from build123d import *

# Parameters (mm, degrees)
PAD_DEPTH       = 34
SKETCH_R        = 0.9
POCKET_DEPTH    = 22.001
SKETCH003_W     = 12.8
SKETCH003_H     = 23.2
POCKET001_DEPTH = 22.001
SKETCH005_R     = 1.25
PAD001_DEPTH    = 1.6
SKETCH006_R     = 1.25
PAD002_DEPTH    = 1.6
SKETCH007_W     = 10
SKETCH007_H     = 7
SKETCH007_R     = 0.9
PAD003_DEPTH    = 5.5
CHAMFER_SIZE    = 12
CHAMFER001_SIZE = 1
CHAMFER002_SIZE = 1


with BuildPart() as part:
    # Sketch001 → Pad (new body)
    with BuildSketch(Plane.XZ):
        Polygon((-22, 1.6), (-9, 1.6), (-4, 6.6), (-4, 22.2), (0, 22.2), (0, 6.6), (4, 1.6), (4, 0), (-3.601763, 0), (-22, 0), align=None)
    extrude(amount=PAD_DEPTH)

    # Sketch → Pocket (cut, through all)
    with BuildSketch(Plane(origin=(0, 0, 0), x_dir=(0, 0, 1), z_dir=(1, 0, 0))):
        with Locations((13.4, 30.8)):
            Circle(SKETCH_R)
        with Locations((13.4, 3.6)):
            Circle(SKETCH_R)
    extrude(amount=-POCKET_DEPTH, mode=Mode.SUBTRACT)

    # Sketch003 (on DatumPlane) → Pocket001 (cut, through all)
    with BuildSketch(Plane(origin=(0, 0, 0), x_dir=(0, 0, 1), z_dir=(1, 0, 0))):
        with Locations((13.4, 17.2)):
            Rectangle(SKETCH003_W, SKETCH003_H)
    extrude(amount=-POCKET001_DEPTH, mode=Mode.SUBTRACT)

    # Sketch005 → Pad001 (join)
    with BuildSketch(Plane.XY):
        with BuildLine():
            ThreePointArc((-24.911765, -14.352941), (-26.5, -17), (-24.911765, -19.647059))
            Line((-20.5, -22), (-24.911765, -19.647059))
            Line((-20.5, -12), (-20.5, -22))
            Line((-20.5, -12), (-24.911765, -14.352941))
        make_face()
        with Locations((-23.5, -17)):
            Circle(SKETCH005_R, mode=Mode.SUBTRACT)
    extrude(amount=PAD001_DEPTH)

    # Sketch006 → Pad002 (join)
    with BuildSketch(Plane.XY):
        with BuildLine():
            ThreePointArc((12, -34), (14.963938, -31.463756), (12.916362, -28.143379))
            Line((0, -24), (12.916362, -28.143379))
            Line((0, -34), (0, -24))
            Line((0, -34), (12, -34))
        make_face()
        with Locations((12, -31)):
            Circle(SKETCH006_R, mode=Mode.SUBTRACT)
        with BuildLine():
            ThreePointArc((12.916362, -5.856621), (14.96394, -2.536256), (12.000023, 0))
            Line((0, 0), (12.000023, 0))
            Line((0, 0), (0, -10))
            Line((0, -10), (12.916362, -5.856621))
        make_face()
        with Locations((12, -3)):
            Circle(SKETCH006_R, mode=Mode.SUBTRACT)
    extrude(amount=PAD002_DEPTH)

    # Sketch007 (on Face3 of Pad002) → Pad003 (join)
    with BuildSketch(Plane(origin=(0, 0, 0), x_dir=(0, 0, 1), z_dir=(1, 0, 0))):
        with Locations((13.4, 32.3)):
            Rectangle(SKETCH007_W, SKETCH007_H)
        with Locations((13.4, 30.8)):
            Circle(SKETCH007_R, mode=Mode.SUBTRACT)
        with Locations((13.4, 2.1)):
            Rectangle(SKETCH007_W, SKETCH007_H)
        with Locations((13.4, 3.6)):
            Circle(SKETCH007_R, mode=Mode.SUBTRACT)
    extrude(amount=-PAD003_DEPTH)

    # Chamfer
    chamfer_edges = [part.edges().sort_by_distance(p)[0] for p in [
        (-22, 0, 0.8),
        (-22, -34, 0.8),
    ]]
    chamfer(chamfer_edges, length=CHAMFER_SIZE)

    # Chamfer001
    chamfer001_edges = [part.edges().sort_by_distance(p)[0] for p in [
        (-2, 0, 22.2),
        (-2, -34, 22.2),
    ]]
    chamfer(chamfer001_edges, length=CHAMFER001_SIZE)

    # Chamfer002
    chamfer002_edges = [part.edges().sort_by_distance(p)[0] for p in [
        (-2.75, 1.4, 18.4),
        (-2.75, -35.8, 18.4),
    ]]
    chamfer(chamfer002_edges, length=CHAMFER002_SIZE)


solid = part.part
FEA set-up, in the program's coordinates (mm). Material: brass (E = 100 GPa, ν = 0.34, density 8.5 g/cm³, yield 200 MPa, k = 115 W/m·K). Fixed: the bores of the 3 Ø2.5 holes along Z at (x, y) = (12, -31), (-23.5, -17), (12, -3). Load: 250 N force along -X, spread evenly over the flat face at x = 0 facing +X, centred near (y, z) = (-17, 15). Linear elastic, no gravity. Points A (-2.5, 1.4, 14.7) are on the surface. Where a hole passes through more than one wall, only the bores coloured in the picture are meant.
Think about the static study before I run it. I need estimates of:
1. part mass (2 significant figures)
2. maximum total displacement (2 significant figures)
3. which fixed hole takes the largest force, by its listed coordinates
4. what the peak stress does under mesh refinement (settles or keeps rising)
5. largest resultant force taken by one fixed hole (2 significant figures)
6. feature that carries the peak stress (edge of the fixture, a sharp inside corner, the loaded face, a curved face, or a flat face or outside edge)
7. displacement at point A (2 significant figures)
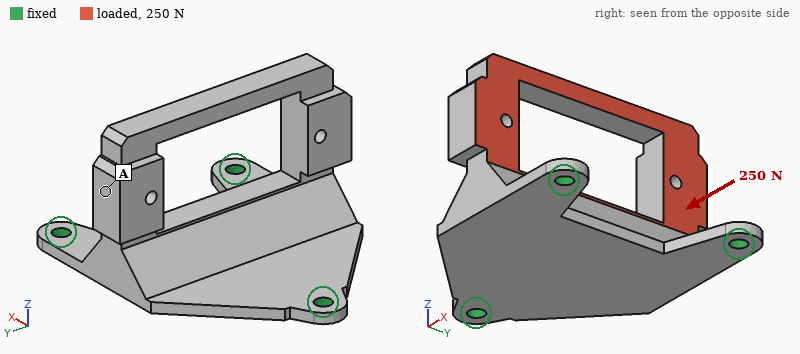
35 g
0.12 mm
(-23.5, -17)
keeps rising
180 N
edge of the fixture
0.067 mm
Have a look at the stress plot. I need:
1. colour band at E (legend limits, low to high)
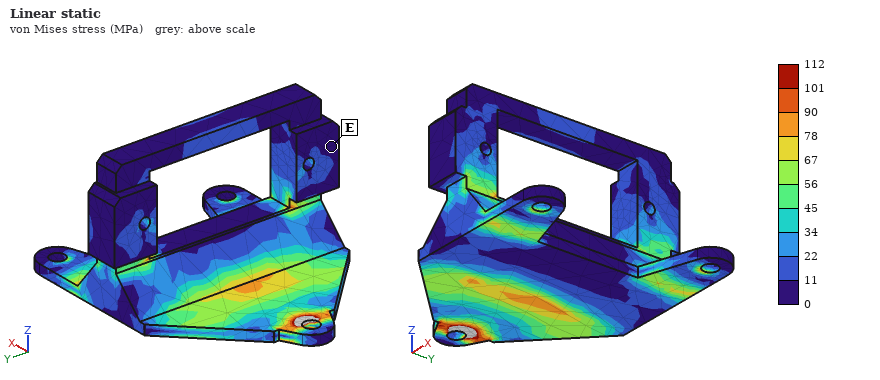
0 to 11 MPa
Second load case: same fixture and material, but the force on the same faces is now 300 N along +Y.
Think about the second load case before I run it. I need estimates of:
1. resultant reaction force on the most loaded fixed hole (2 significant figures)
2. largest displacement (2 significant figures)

200 N
0.10 mm
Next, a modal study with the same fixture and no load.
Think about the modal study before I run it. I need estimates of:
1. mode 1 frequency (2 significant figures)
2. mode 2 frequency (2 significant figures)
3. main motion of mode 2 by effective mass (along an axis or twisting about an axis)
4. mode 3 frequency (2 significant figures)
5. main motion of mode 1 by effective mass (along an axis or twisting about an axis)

2100 Hz
2400 Hz
along Y
3700 Hz
along Z
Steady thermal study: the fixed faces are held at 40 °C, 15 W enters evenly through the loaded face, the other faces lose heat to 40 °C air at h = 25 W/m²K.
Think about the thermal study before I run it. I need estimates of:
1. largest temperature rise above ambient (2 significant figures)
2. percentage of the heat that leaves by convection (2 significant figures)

63 K
15 %
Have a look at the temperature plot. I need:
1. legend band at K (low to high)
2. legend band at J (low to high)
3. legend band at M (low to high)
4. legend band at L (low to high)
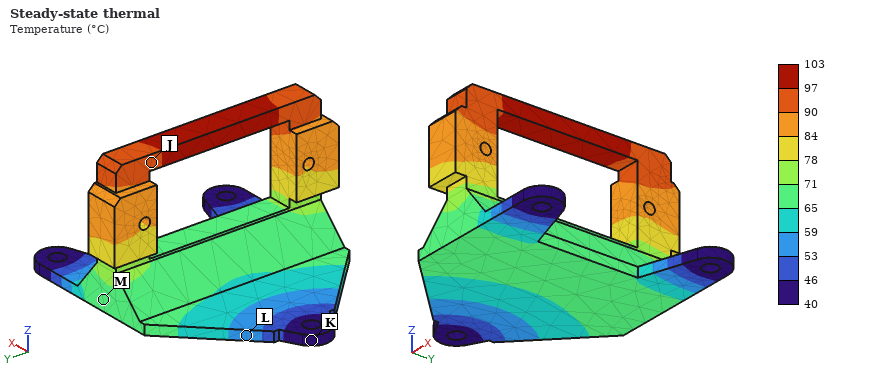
40 to 46 °C
90 to 97 °C
65 to 71 °C
53 to 59 °C
